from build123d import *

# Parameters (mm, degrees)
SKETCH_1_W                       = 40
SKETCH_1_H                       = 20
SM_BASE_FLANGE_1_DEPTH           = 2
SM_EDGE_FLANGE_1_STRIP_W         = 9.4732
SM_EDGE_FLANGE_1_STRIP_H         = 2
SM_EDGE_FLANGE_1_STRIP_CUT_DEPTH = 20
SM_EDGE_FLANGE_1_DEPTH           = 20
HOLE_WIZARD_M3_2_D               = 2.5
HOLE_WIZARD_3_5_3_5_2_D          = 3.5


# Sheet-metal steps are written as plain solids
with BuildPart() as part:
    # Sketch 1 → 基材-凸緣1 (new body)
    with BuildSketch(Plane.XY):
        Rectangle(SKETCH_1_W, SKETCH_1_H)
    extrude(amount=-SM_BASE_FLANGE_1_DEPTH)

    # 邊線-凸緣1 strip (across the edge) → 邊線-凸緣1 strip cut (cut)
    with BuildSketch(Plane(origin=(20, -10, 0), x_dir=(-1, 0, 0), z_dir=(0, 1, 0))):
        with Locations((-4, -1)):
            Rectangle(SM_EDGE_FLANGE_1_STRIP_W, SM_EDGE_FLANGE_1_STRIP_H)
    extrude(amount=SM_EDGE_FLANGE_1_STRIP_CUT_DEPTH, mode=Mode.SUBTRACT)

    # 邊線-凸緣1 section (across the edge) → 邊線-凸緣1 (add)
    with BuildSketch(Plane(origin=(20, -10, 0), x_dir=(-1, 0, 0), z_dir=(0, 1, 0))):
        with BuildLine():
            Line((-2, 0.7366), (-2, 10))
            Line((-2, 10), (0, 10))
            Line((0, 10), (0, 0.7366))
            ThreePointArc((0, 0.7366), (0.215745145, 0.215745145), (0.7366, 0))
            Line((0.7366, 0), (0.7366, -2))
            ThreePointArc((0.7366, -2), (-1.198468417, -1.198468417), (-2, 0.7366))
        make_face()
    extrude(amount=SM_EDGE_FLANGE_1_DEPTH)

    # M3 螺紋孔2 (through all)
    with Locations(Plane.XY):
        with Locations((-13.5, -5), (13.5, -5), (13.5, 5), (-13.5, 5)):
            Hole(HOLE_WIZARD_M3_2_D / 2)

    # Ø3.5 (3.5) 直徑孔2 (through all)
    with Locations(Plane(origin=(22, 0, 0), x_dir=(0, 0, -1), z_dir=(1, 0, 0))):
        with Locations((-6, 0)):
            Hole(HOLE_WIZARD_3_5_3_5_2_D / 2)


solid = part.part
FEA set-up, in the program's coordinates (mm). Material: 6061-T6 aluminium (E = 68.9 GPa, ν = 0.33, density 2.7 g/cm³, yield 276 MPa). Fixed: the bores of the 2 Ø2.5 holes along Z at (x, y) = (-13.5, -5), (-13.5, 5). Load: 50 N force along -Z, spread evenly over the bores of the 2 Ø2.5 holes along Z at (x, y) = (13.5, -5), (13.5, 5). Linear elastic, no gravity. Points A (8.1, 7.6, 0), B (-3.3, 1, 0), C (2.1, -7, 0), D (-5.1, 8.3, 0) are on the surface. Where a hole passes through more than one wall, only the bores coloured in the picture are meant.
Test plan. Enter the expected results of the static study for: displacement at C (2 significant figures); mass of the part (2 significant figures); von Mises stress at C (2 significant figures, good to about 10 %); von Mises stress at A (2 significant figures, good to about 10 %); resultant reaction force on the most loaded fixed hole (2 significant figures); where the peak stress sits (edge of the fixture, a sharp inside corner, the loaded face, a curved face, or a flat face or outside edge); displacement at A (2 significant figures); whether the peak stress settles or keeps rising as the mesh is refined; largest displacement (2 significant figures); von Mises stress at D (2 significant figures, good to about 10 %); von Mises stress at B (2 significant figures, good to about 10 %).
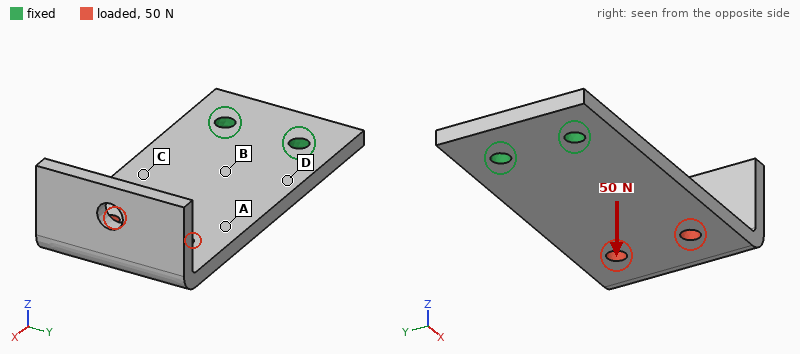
0.13 mm
5.4 g
42 MPa
21 MPa
25 N
edge of the fixture
0.23 mm
keeps rising
0.53 mm
69 MPa
58 MPa
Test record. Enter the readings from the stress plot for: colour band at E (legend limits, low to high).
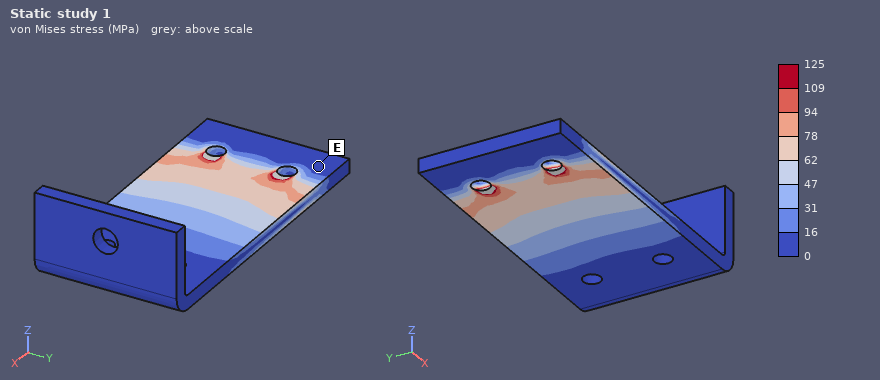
0 to 16 MPa
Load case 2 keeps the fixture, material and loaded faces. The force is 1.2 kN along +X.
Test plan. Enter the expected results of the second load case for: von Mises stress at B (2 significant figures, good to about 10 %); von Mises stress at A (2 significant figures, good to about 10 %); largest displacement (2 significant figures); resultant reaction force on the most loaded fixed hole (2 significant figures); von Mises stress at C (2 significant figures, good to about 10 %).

31 MPa
30 MPa
14 µm
600 N
30 MPa
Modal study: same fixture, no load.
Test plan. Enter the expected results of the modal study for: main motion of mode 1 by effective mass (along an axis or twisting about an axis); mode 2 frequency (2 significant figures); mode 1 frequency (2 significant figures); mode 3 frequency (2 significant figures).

along Z
3000 Hz
950 Hz
5100 Hz
